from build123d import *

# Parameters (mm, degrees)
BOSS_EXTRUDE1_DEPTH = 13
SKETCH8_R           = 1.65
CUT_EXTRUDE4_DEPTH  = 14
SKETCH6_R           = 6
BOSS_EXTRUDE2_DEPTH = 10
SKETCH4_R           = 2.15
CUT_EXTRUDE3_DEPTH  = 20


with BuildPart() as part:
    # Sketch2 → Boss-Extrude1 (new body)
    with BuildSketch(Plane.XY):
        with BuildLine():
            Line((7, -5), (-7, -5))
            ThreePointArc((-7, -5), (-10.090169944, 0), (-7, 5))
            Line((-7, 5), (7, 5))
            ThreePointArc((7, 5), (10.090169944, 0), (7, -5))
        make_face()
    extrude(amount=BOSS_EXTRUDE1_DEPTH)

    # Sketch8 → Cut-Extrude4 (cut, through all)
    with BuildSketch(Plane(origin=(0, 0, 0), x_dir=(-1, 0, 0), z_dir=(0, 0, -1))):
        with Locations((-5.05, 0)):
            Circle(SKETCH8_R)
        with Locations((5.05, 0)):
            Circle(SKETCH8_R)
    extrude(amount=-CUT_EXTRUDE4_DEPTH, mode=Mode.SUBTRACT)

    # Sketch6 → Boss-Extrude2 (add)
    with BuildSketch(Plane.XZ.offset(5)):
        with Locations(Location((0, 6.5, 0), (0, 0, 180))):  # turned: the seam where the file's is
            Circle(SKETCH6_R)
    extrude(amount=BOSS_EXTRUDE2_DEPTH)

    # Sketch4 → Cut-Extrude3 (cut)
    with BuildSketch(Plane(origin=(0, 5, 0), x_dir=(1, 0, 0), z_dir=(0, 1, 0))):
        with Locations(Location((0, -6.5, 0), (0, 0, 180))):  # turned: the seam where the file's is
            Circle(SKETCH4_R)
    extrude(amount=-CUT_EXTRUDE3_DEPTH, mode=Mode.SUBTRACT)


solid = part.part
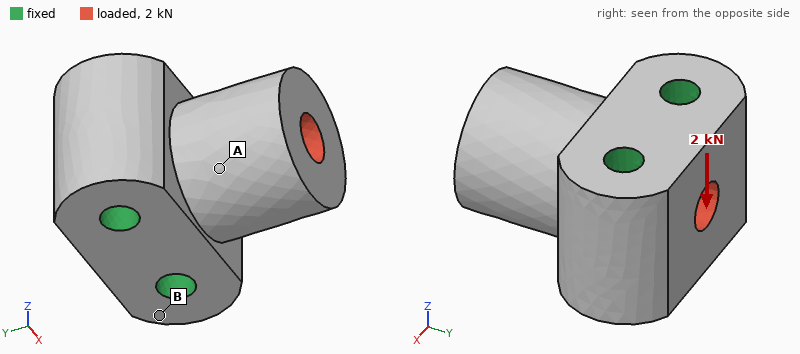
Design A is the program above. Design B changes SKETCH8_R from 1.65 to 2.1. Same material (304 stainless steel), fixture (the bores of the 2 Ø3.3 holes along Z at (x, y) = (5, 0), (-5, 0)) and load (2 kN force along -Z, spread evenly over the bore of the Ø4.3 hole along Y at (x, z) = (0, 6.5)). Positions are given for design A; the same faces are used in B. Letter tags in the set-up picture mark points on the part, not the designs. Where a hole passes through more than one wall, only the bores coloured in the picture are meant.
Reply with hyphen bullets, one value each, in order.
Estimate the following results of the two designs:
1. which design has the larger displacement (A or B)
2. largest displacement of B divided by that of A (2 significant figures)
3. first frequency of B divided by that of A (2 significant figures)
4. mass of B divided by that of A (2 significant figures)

- A
- 0.92
- 1.0
- 0.95
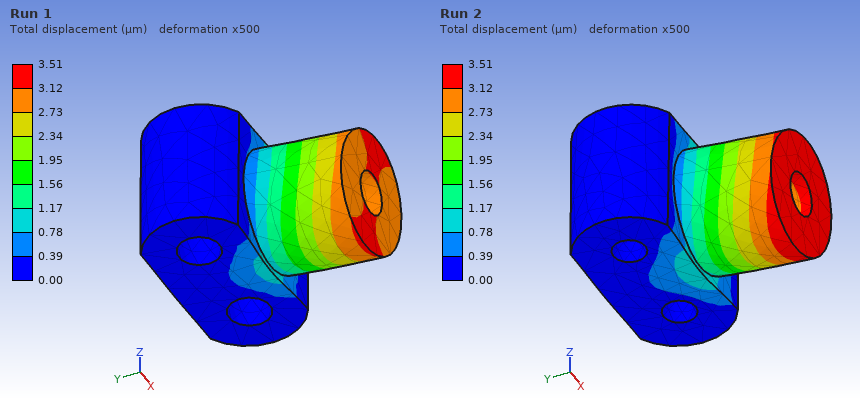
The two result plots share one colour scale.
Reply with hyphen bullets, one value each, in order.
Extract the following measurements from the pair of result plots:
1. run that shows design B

- Run 1
